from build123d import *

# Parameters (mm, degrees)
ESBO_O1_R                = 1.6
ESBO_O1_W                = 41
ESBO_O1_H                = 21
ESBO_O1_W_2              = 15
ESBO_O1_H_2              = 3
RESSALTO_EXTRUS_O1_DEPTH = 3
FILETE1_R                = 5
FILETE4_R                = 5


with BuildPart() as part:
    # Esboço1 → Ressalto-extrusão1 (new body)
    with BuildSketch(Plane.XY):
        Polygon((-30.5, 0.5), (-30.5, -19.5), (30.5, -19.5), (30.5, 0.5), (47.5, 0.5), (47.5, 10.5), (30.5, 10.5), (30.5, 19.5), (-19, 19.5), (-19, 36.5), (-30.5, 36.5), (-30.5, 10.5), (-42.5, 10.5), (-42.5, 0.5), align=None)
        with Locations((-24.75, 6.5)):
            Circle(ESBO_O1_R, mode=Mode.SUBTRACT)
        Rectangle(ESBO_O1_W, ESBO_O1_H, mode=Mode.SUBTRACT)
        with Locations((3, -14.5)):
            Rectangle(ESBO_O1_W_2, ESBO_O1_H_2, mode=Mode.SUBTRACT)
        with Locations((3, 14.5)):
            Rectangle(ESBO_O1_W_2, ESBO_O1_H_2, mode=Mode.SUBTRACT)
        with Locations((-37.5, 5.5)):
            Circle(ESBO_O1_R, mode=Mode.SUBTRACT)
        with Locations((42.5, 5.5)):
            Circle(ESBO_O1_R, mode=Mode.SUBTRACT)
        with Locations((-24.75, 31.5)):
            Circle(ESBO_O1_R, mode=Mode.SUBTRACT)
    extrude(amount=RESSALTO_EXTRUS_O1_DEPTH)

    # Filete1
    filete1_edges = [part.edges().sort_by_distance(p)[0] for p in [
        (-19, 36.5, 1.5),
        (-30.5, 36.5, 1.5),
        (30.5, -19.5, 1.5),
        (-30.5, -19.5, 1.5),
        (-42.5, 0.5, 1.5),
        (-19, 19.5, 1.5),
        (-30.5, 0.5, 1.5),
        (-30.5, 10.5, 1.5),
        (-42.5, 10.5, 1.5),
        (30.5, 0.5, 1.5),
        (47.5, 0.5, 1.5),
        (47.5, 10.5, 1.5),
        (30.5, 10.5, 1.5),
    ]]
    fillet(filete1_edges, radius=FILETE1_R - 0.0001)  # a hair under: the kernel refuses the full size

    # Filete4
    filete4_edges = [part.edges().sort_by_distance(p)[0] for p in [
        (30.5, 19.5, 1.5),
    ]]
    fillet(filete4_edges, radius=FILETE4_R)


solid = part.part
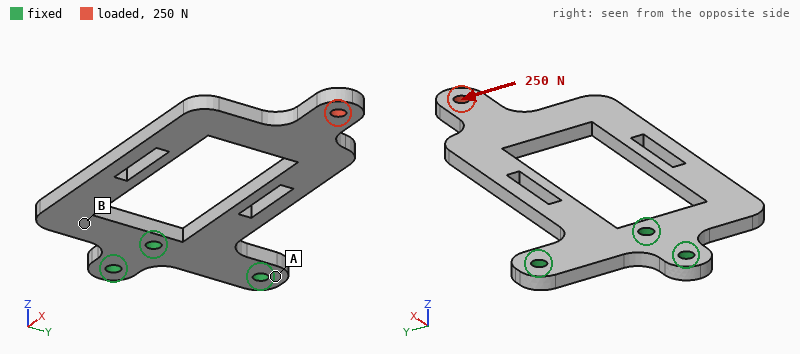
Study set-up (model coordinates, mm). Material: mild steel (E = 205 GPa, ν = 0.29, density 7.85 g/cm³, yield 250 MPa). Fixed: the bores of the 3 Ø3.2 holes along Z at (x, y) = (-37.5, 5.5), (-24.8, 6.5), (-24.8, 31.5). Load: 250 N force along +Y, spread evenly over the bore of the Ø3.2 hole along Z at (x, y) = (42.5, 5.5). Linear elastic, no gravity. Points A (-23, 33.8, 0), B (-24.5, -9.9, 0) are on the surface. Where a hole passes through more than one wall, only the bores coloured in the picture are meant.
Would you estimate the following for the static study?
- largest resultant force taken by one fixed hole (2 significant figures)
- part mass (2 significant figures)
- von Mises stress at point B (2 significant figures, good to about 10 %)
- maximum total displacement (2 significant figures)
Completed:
670 N
44 g
32 MPa
0.12 mm
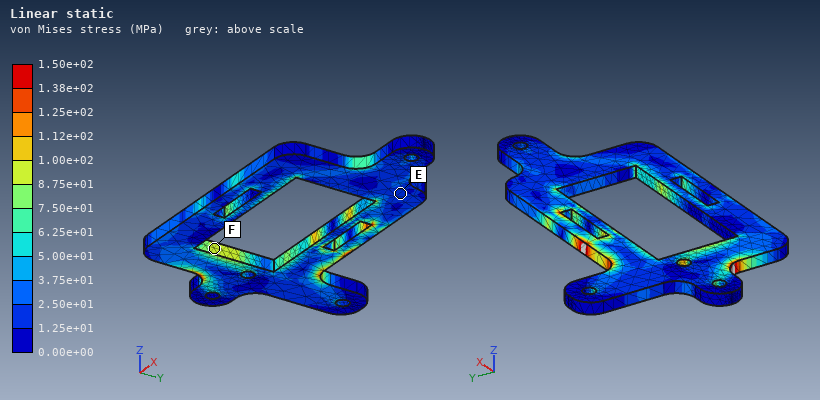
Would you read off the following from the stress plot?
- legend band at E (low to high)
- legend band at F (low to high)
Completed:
1.25e+01 to 2.50e+01 MPa
8.75e+01 to 1.00e+02 MPa
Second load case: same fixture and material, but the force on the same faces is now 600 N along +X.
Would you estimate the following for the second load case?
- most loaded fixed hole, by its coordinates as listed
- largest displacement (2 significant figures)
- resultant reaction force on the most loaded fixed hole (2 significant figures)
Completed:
(-24.8, 6.5)
21 µm
340 N
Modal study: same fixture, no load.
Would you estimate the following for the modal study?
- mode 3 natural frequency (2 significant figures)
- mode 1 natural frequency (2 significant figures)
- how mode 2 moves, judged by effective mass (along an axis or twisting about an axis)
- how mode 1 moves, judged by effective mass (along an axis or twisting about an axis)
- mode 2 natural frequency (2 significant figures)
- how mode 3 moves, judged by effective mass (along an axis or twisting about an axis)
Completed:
2000 Hz
440 Hz
twisting about X
along Z
1400 Hz
along Y
